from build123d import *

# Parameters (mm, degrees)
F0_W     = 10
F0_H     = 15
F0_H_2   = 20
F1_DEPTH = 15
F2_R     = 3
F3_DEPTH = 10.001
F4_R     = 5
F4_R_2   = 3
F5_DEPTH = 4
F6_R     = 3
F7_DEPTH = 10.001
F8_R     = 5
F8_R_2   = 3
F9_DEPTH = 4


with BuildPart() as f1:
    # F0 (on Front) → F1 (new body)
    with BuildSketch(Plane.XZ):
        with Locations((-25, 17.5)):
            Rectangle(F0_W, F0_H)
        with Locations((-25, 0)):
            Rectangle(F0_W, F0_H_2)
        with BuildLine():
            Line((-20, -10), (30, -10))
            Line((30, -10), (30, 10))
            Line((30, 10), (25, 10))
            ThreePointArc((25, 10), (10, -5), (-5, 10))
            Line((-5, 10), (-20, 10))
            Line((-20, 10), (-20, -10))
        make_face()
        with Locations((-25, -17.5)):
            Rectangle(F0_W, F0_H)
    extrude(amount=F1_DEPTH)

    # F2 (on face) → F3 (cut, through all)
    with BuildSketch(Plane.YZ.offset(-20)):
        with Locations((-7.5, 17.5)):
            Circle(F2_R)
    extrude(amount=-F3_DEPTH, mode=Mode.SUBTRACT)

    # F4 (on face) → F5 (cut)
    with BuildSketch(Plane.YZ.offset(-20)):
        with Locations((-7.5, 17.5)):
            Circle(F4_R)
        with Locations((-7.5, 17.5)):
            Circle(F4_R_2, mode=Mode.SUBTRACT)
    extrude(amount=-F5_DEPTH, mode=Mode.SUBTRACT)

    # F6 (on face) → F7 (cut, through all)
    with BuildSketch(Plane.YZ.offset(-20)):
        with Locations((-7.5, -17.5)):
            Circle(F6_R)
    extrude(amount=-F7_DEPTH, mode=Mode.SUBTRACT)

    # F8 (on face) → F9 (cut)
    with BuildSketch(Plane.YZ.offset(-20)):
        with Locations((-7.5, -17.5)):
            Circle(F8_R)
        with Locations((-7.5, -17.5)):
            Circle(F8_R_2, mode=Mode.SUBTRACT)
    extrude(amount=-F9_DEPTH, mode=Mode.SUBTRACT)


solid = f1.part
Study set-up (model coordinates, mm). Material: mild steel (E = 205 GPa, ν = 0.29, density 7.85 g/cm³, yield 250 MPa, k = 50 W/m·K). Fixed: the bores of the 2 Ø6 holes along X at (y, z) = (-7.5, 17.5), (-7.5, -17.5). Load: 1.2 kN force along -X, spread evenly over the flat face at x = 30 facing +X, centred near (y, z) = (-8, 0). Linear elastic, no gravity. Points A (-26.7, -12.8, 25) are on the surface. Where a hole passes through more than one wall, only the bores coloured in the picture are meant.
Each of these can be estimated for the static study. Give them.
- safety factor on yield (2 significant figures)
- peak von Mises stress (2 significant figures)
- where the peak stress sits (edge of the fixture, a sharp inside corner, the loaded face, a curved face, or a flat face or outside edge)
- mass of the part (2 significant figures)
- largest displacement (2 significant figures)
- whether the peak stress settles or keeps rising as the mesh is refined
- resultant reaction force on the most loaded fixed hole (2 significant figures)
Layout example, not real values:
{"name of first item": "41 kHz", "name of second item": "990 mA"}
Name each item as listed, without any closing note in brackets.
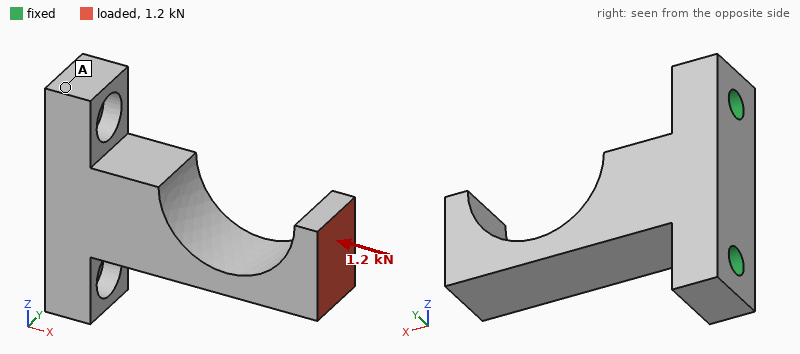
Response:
{"safety factor on yield": "1.6", "peak von Mises stress": "160 MPa", "where the peak stress sits": "a curved face", "mass of the part": "130 g", "largest displacement": "0.11 mm", "whether the peak stress settles or keeps rising as the mesh is refined": "settles", "resultant reaction force on the most loaded fixed hole": "680 N"}
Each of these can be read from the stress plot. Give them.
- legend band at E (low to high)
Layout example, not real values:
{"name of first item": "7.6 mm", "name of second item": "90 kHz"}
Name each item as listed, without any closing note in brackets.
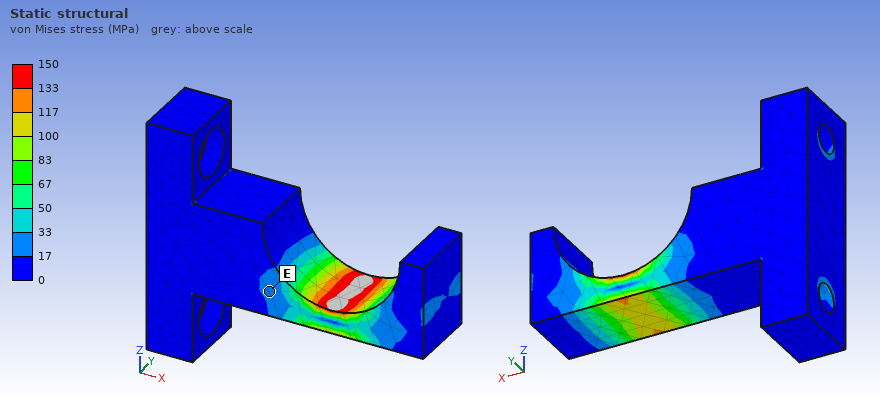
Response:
{"legend band at E": "17 to 33 MPa"}
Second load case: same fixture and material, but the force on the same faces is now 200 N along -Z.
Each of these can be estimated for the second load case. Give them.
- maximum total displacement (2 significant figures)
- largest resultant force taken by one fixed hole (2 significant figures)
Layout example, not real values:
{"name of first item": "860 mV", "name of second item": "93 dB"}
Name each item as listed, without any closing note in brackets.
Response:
{"maximum total displacement": "58 µm", "largest resultant force taken by one fixed hole": "410 N"}
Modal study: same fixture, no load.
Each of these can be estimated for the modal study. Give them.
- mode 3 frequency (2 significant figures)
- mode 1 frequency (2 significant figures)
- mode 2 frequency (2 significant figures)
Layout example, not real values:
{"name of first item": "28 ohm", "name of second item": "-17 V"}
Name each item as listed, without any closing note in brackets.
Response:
{"mode 3 frequency": "7600 Hz", "mode 1 frequency": "2500 Hz", "mode 2 frequency": "2500 Hz"}
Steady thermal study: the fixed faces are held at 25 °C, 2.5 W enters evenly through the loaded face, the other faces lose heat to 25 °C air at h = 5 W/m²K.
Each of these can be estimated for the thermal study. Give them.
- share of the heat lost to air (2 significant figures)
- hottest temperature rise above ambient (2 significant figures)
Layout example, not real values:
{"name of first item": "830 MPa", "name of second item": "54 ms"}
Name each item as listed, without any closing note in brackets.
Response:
{"share of the heat lost to air": "6.7 %", "hottest temperature rise above ambient": "22 K"}
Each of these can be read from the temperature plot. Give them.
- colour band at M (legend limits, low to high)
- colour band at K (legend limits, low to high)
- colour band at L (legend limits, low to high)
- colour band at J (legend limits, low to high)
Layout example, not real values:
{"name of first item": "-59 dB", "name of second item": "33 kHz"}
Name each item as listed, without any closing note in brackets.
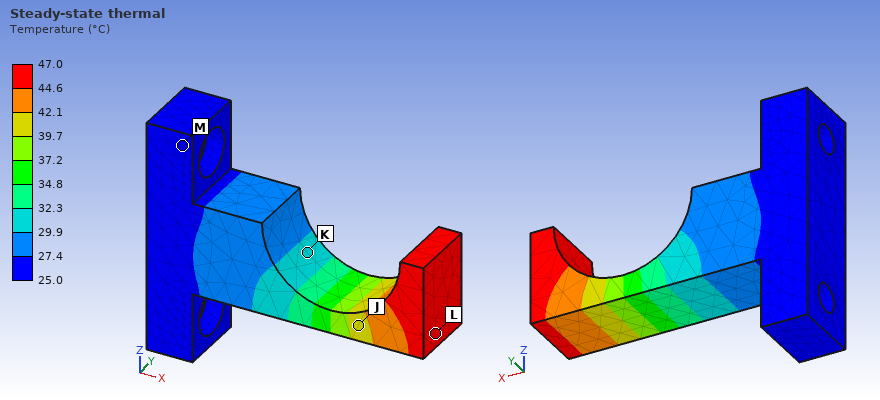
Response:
{"colour band at M": "25.0 to 27.4 °C", "colour band at K": "29.9 to 32.3 °C", "colour band at L": "44.6 to 47.0 °C", "colour band at J": "39.7 to 42.1 °C"}
